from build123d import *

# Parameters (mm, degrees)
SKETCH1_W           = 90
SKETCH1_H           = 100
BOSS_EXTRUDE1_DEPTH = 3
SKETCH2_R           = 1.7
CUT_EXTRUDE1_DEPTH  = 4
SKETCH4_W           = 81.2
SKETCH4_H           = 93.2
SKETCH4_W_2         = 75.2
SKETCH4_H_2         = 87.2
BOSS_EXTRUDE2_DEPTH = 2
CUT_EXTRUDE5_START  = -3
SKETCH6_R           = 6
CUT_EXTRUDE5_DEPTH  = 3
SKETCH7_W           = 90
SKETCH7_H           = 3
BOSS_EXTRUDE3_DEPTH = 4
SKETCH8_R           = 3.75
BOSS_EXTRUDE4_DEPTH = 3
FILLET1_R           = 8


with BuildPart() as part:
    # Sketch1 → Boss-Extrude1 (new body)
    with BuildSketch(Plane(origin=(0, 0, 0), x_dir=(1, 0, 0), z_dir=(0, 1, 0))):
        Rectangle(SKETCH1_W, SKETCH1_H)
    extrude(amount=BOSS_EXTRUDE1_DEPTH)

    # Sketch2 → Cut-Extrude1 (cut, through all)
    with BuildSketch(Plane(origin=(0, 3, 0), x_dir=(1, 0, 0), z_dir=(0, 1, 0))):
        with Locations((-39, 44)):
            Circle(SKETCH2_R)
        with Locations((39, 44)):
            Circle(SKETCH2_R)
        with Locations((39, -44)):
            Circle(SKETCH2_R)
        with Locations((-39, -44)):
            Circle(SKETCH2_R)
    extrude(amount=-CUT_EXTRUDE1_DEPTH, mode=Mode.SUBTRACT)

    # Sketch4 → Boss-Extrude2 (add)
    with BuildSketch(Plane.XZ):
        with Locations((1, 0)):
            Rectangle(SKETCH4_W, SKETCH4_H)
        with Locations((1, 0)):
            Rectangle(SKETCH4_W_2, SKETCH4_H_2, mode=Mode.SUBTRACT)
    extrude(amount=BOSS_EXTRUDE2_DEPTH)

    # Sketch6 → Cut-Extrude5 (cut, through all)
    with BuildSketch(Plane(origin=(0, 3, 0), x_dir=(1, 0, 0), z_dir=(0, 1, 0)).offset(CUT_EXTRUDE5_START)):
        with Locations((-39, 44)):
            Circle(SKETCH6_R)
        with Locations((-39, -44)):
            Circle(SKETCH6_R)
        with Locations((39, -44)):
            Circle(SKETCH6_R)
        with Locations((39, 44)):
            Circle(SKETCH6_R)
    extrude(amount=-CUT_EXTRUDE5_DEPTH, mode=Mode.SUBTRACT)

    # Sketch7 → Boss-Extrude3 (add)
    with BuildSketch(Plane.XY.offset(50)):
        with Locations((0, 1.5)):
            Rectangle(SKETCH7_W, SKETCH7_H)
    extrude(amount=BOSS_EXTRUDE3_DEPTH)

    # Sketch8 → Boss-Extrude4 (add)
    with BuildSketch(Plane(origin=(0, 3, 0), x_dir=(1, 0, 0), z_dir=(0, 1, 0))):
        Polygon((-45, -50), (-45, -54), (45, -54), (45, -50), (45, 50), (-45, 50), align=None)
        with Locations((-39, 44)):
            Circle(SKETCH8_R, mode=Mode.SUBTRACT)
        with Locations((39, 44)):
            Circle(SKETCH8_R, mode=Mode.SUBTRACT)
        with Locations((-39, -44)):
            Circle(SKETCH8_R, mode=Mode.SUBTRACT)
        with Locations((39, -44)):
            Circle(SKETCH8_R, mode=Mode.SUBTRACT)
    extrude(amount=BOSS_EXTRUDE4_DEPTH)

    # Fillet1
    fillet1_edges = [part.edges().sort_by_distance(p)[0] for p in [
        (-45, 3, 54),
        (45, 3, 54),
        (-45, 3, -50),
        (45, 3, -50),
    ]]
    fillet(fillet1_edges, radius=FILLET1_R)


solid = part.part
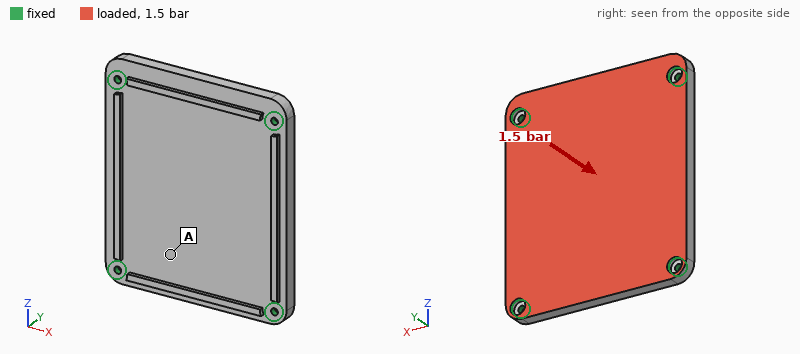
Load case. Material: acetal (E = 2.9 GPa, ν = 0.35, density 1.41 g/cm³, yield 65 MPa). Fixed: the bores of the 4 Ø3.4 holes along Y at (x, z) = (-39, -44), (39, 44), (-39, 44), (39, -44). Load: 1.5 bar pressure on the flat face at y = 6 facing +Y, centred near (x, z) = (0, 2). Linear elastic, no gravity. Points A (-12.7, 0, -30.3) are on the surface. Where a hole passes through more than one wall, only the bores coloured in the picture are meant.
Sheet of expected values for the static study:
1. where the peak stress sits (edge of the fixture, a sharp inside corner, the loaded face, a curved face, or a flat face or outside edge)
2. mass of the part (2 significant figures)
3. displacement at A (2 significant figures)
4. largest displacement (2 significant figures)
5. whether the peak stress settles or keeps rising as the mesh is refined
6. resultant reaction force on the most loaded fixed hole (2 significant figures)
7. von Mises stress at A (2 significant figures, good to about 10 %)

edge of the fixture
80 g
0.96 mm
1.5 mm
keeps rising
580 N
7.4 MPa
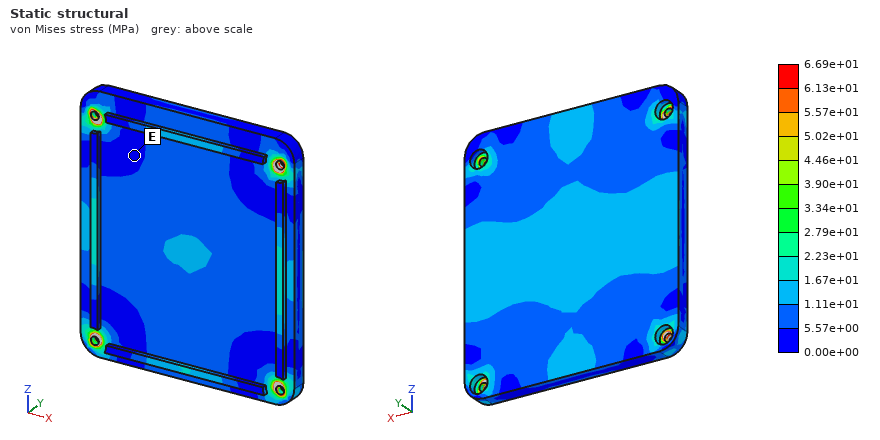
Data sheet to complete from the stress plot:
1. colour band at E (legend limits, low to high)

0.00e+00 to 5.57e+00 MPa
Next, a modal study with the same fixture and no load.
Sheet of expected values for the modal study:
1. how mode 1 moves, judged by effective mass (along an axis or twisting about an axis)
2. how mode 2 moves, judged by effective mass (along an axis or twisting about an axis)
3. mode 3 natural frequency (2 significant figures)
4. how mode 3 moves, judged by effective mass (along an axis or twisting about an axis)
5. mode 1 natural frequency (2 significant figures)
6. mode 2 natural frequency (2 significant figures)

along Y
twisting about Z
1200 Hz
twisting about X
650 Hz
1100 Hz
